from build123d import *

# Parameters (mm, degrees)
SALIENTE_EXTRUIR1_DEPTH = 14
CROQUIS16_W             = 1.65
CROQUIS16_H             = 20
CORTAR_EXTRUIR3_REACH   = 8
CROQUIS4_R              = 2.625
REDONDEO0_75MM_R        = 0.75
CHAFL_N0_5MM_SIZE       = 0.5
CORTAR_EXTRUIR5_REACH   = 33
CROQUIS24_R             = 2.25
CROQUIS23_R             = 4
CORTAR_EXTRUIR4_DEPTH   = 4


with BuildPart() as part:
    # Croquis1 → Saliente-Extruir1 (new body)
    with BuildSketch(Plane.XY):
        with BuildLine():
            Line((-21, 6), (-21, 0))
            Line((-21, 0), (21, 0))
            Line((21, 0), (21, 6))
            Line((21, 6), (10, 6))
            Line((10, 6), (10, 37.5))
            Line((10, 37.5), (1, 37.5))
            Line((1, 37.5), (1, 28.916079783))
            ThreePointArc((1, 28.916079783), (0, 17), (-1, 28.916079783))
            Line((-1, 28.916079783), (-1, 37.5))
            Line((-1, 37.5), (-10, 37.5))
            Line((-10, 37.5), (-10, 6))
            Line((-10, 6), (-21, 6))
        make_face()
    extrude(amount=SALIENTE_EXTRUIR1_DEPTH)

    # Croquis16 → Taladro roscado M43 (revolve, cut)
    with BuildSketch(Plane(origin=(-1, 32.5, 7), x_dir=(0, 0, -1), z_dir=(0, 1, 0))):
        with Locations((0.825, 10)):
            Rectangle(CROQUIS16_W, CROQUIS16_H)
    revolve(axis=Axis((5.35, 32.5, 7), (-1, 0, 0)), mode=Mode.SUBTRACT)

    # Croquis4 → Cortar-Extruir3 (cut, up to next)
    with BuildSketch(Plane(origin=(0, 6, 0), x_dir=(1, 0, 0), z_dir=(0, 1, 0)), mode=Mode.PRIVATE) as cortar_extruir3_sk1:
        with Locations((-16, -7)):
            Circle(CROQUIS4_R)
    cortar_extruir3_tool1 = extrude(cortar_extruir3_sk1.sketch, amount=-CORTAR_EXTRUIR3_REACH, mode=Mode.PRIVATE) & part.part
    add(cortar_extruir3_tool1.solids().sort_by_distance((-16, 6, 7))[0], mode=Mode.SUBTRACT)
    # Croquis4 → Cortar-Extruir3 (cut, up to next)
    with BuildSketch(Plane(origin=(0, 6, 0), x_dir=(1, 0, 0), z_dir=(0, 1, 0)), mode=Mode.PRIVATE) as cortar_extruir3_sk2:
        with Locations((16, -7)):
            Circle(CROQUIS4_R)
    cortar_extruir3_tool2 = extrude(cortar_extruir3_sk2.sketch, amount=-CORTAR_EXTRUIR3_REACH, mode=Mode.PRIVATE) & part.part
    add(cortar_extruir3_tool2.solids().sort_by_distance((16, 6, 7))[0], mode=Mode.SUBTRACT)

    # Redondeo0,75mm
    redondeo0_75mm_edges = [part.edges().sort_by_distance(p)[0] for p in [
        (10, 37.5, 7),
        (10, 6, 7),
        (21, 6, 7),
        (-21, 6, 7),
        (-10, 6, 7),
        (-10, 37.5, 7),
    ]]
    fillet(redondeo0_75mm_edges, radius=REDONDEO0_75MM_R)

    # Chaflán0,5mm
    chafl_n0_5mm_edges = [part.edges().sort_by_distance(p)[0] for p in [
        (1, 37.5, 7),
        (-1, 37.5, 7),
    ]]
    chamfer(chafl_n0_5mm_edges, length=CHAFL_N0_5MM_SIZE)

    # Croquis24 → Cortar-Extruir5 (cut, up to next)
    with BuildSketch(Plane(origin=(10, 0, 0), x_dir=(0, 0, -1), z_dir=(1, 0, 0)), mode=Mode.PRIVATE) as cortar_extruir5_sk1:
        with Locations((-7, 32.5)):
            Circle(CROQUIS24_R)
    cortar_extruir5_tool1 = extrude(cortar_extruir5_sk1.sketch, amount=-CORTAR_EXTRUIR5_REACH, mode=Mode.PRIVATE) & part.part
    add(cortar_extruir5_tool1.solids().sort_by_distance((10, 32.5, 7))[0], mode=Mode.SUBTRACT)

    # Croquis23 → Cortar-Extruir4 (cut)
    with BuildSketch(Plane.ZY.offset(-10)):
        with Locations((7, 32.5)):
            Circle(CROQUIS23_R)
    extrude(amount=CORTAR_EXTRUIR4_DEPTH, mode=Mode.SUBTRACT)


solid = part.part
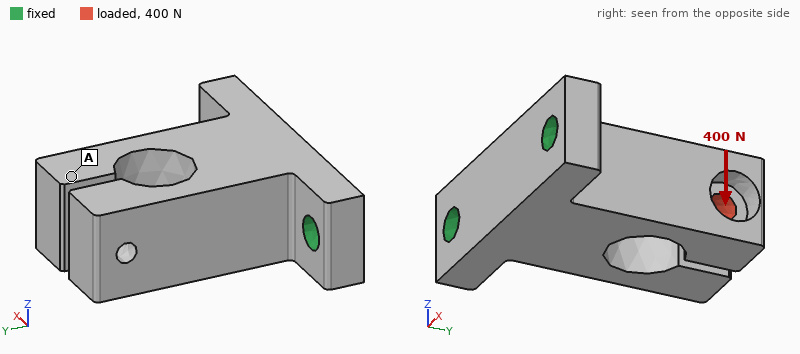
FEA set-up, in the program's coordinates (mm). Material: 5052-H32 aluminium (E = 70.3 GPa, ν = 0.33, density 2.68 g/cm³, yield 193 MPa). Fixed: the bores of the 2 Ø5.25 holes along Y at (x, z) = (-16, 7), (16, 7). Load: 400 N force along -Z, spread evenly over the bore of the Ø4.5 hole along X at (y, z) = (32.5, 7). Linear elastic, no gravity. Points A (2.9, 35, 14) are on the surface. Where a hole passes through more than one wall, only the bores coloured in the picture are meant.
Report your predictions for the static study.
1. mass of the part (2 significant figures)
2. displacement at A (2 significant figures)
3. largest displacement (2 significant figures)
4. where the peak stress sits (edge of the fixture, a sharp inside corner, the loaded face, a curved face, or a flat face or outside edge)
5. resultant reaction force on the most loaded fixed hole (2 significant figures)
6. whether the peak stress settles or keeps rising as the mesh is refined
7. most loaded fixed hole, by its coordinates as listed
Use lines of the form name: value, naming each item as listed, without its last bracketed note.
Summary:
mass of the part: 27 g
displacement at A: 0.093 mm
largest displacement: 0.10 mm
where the peak stress sits: edge of the fixture
resultant reaction force on the most loaded fixed hole: 240 N
whether the peak stress settles or keeps rising as the mesh is refined: keeps rising
most loaded fixed hole, by its coordinates as listed: (16, 7)
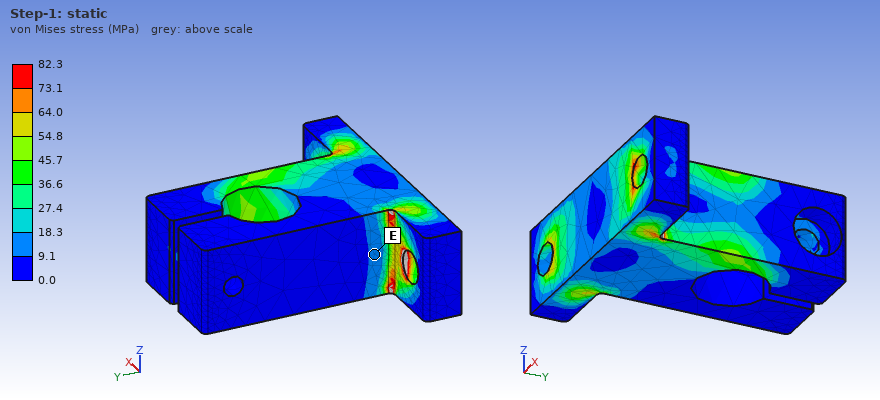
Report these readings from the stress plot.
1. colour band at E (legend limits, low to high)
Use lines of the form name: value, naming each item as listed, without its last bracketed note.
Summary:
colour band at E: 9.1 to 18.3 MPa
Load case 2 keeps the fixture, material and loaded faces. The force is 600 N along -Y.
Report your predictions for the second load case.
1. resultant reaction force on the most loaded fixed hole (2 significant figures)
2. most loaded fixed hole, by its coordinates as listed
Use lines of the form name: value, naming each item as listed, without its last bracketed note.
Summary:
resultant reaction force on the most loaded fixed hole: 410 N
most loaded fixed hole, by its coordinates as listed: (16, 7)
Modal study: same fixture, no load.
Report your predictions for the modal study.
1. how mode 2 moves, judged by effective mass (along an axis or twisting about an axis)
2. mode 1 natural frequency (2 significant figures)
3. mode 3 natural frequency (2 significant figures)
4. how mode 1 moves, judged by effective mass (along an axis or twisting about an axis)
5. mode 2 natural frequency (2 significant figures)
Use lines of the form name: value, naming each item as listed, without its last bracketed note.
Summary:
how mode 2 moves, judged by effective mass: along X
mode 1 natural frequency: 4400 Hz
mode 3 natural frequency: 6300 Hz
how mode 1 moves, judged by effective mass: along Z
mode 2 natural frequency: 5600 Hz
